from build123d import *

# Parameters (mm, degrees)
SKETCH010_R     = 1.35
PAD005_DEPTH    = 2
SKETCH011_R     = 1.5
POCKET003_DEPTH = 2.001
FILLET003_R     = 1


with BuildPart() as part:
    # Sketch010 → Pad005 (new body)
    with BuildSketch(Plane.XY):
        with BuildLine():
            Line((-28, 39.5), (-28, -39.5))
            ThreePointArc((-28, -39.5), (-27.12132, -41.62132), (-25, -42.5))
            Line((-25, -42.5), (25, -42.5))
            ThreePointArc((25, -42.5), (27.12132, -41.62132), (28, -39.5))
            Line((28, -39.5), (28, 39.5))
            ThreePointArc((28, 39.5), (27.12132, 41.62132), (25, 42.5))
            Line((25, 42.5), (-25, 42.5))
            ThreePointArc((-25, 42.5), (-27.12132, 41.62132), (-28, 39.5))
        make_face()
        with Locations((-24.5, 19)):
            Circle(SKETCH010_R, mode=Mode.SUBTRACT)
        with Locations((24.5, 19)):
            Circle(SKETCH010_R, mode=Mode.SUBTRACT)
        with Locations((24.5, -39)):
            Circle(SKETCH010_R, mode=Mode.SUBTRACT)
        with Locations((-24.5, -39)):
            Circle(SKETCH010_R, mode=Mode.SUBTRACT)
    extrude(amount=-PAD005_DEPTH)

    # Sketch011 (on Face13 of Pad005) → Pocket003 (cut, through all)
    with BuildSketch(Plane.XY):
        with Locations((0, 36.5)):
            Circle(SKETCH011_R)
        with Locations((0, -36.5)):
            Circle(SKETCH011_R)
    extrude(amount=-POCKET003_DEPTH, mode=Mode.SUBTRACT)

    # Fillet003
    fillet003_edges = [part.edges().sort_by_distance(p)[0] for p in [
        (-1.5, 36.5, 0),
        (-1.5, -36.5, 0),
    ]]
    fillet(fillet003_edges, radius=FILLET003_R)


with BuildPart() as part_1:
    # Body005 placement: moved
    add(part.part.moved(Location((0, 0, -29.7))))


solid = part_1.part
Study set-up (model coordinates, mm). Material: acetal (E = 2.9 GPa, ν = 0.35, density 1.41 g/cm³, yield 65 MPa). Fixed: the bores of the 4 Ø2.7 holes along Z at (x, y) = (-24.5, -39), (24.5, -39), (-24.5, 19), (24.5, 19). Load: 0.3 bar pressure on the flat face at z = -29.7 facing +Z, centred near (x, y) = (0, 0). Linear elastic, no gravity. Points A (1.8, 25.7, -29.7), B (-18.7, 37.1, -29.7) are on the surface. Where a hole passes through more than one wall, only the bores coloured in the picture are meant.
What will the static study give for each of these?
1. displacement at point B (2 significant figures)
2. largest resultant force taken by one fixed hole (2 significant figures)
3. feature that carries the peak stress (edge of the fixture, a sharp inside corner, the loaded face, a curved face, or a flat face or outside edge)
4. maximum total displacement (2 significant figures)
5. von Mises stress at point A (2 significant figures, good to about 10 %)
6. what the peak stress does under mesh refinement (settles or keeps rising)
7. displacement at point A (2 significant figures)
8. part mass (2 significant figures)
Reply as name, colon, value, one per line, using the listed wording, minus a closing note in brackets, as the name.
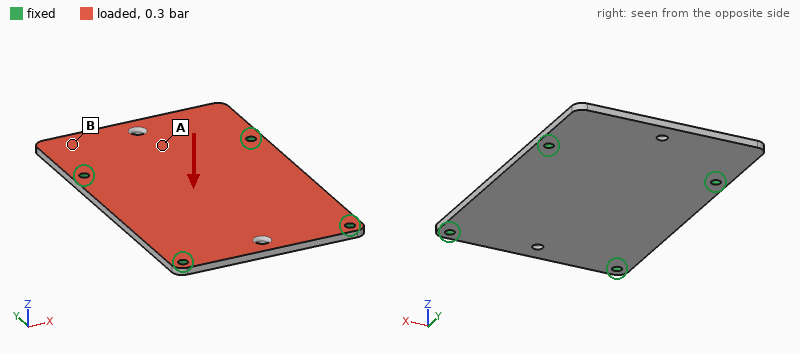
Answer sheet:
displacement at point B: 0.52 mm
largest resultant force taken by one fixed hole: 45 N
feature that carries the peak stress: edge of the fixture
maximum total displacement: 0.94 mm
von Mises stress at point A: 8.1 MPa
what the peak stress does under mesh refinement: keeps rising
displacement at point A: 0.52 mm
part mass: 13 g
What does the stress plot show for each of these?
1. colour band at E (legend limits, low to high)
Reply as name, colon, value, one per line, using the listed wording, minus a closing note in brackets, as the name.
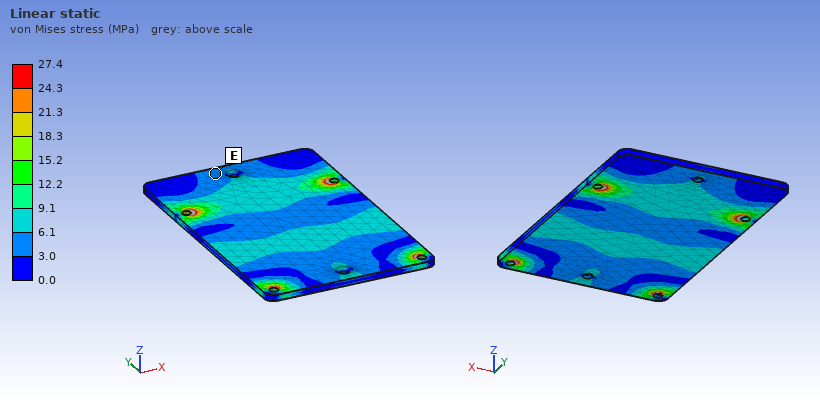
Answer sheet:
colour band at E: 3.0 to 6.1 MPa
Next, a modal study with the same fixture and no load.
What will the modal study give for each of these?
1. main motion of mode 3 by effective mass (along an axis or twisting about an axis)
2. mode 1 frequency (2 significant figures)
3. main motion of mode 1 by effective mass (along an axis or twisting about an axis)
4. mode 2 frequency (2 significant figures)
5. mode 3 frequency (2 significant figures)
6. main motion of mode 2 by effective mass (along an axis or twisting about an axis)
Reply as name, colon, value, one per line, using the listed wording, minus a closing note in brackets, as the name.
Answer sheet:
main motion of mode 3 by effective mass: twisting about Y
mode 1 frequency: 590 Hz
main motion of mode 1 by effective mass: twisting about X
mode 2 frequency: 680 Hz
mode 3 frequency: 1000 Hz
main motion of mode 2 by effective mass: along Z
